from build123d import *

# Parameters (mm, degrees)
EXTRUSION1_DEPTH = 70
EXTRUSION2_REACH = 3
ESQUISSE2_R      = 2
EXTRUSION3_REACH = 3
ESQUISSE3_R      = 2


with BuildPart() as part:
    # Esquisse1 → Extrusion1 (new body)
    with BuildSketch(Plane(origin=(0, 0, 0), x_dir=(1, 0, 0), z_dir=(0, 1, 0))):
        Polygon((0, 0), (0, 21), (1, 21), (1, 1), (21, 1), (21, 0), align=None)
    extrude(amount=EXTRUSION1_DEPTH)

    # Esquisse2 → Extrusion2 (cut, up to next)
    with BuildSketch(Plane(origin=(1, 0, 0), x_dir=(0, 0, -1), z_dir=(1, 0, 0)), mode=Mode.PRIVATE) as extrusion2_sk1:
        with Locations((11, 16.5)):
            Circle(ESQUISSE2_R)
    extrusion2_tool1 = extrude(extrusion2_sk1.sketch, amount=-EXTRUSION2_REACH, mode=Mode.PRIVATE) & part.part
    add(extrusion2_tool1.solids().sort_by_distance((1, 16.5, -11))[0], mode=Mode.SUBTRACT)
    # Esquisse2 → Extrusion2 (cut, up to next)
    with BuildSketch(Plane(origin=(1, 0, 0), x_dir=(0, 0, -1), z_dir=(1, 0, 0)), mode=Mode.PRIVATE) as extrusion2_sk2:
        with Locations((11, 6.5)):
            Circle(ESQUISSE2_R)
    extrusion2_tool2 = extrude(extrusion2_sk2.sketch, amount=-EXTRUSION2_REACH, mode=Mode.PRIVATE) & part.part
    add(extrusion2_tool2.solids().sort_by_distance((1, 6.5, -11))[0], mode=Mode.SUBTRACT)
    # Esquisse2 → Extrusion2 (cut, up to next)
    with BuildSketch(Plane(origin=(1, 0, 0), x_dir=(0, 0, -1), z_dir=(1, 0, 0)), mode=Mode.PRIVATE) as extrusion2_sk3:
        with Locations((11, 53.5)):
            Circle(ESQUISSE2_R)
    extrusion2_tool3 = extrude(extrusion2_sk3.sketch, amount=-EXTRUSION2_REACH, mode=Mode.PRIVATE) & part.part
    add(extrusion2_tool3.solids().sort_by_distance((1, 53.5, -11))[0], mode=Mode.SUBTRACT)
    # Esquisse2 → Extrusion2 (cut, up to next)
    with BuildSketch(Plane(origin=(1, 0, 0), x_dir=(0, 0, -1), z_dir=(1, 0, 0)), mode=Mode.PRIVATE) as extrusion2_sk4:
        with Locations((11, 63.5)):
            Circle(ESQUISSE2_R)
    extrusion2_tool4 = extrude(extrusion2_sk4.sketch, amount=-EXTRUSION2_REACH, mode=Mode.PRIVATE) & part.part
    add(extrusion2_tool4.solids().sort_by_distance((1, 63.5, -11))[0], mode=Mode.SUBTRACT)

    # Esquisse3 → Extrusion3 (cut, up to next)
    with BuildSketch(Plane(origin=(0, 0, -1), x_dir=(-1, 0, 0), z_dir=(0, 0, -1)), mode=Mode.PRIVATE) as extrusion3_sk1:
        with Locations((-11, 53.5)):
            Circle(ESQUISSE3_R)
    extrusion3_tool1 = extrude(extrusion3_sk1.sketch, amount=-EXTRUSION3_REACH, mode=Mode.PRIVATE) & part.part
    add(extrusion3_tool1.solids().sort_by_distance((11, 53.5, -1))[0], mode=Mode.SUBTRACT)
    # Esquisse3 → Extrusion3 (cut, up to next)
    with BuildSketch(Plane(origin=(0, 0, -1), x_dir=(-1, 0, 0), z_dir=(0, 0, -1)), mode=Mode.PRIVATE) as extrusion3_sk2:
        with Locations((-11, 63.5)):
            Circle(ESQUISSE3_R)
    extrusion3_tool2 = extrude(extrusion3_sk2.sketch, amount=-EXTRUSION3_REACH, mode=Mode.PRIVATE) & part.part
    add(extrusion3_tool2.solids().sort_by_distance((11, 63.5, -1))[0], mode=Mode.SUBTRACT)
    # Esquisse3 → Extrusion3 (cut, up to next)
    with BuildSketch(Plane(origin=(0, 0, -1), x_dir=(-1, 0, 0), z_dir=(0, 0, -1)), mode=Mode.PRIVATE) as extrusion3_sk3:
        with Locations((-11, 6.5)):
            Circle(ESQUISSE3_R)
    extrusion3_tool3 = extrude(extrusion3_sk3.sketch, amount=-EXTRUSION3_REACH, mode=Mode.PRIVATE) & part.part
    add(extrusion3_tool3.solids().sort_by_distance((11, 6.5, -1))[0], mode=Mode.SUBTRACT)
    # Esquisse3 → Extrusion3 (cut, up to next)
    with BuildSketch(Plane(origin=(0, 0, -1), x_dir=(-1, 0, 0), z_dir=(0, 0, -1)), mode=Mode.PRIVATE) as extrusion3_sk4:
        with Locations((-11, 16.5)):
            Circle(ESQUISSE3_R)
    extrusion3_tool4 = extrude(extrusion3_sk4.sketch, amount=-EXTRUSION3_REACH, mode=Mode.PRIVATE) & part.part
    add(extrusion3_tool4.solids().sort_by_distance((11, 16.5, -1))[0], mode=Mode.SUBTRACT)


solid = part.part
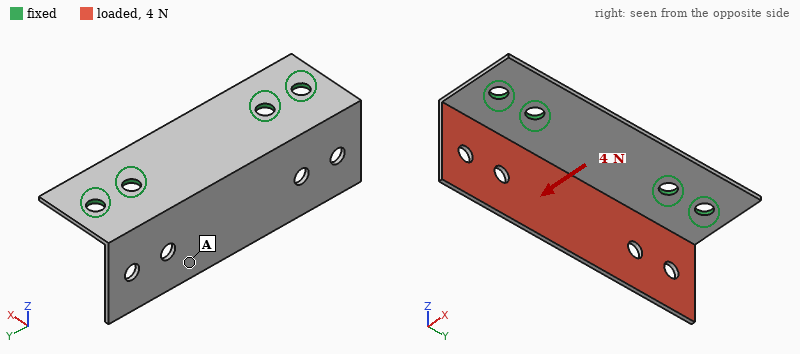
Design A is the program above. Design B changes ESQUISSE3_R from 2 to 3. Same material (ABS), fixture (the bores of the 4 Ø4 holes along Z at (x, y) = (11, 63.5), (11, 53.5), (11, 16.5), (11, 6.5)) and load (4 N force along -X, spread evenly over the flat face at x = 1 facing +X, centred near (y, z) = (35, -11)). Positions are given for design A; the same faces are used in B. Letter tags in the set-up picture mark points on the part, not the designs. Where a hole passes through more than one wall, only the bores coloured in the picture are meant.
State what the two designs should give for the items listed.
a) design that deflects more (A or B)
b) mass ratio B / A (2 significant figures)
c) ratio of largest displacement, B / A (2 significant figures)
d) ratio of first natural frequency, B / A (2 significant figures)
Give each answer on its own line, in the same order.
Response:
A
0.98
0.90
1.1
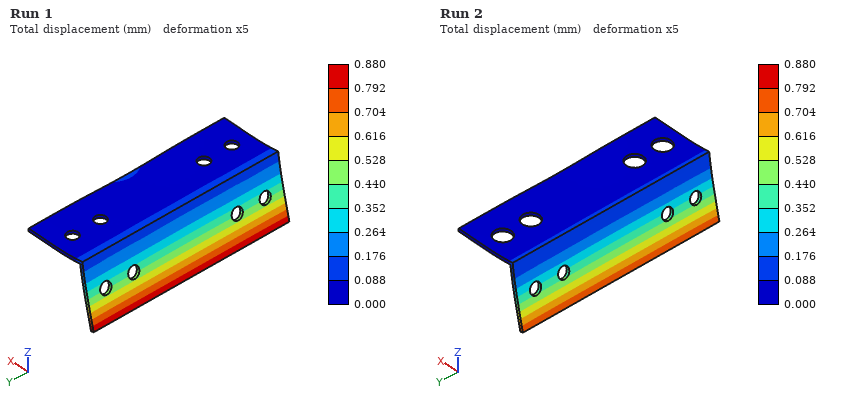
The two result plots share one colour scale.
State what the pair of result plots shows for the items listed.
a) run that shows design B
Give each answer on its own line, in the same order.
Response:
Run 2
